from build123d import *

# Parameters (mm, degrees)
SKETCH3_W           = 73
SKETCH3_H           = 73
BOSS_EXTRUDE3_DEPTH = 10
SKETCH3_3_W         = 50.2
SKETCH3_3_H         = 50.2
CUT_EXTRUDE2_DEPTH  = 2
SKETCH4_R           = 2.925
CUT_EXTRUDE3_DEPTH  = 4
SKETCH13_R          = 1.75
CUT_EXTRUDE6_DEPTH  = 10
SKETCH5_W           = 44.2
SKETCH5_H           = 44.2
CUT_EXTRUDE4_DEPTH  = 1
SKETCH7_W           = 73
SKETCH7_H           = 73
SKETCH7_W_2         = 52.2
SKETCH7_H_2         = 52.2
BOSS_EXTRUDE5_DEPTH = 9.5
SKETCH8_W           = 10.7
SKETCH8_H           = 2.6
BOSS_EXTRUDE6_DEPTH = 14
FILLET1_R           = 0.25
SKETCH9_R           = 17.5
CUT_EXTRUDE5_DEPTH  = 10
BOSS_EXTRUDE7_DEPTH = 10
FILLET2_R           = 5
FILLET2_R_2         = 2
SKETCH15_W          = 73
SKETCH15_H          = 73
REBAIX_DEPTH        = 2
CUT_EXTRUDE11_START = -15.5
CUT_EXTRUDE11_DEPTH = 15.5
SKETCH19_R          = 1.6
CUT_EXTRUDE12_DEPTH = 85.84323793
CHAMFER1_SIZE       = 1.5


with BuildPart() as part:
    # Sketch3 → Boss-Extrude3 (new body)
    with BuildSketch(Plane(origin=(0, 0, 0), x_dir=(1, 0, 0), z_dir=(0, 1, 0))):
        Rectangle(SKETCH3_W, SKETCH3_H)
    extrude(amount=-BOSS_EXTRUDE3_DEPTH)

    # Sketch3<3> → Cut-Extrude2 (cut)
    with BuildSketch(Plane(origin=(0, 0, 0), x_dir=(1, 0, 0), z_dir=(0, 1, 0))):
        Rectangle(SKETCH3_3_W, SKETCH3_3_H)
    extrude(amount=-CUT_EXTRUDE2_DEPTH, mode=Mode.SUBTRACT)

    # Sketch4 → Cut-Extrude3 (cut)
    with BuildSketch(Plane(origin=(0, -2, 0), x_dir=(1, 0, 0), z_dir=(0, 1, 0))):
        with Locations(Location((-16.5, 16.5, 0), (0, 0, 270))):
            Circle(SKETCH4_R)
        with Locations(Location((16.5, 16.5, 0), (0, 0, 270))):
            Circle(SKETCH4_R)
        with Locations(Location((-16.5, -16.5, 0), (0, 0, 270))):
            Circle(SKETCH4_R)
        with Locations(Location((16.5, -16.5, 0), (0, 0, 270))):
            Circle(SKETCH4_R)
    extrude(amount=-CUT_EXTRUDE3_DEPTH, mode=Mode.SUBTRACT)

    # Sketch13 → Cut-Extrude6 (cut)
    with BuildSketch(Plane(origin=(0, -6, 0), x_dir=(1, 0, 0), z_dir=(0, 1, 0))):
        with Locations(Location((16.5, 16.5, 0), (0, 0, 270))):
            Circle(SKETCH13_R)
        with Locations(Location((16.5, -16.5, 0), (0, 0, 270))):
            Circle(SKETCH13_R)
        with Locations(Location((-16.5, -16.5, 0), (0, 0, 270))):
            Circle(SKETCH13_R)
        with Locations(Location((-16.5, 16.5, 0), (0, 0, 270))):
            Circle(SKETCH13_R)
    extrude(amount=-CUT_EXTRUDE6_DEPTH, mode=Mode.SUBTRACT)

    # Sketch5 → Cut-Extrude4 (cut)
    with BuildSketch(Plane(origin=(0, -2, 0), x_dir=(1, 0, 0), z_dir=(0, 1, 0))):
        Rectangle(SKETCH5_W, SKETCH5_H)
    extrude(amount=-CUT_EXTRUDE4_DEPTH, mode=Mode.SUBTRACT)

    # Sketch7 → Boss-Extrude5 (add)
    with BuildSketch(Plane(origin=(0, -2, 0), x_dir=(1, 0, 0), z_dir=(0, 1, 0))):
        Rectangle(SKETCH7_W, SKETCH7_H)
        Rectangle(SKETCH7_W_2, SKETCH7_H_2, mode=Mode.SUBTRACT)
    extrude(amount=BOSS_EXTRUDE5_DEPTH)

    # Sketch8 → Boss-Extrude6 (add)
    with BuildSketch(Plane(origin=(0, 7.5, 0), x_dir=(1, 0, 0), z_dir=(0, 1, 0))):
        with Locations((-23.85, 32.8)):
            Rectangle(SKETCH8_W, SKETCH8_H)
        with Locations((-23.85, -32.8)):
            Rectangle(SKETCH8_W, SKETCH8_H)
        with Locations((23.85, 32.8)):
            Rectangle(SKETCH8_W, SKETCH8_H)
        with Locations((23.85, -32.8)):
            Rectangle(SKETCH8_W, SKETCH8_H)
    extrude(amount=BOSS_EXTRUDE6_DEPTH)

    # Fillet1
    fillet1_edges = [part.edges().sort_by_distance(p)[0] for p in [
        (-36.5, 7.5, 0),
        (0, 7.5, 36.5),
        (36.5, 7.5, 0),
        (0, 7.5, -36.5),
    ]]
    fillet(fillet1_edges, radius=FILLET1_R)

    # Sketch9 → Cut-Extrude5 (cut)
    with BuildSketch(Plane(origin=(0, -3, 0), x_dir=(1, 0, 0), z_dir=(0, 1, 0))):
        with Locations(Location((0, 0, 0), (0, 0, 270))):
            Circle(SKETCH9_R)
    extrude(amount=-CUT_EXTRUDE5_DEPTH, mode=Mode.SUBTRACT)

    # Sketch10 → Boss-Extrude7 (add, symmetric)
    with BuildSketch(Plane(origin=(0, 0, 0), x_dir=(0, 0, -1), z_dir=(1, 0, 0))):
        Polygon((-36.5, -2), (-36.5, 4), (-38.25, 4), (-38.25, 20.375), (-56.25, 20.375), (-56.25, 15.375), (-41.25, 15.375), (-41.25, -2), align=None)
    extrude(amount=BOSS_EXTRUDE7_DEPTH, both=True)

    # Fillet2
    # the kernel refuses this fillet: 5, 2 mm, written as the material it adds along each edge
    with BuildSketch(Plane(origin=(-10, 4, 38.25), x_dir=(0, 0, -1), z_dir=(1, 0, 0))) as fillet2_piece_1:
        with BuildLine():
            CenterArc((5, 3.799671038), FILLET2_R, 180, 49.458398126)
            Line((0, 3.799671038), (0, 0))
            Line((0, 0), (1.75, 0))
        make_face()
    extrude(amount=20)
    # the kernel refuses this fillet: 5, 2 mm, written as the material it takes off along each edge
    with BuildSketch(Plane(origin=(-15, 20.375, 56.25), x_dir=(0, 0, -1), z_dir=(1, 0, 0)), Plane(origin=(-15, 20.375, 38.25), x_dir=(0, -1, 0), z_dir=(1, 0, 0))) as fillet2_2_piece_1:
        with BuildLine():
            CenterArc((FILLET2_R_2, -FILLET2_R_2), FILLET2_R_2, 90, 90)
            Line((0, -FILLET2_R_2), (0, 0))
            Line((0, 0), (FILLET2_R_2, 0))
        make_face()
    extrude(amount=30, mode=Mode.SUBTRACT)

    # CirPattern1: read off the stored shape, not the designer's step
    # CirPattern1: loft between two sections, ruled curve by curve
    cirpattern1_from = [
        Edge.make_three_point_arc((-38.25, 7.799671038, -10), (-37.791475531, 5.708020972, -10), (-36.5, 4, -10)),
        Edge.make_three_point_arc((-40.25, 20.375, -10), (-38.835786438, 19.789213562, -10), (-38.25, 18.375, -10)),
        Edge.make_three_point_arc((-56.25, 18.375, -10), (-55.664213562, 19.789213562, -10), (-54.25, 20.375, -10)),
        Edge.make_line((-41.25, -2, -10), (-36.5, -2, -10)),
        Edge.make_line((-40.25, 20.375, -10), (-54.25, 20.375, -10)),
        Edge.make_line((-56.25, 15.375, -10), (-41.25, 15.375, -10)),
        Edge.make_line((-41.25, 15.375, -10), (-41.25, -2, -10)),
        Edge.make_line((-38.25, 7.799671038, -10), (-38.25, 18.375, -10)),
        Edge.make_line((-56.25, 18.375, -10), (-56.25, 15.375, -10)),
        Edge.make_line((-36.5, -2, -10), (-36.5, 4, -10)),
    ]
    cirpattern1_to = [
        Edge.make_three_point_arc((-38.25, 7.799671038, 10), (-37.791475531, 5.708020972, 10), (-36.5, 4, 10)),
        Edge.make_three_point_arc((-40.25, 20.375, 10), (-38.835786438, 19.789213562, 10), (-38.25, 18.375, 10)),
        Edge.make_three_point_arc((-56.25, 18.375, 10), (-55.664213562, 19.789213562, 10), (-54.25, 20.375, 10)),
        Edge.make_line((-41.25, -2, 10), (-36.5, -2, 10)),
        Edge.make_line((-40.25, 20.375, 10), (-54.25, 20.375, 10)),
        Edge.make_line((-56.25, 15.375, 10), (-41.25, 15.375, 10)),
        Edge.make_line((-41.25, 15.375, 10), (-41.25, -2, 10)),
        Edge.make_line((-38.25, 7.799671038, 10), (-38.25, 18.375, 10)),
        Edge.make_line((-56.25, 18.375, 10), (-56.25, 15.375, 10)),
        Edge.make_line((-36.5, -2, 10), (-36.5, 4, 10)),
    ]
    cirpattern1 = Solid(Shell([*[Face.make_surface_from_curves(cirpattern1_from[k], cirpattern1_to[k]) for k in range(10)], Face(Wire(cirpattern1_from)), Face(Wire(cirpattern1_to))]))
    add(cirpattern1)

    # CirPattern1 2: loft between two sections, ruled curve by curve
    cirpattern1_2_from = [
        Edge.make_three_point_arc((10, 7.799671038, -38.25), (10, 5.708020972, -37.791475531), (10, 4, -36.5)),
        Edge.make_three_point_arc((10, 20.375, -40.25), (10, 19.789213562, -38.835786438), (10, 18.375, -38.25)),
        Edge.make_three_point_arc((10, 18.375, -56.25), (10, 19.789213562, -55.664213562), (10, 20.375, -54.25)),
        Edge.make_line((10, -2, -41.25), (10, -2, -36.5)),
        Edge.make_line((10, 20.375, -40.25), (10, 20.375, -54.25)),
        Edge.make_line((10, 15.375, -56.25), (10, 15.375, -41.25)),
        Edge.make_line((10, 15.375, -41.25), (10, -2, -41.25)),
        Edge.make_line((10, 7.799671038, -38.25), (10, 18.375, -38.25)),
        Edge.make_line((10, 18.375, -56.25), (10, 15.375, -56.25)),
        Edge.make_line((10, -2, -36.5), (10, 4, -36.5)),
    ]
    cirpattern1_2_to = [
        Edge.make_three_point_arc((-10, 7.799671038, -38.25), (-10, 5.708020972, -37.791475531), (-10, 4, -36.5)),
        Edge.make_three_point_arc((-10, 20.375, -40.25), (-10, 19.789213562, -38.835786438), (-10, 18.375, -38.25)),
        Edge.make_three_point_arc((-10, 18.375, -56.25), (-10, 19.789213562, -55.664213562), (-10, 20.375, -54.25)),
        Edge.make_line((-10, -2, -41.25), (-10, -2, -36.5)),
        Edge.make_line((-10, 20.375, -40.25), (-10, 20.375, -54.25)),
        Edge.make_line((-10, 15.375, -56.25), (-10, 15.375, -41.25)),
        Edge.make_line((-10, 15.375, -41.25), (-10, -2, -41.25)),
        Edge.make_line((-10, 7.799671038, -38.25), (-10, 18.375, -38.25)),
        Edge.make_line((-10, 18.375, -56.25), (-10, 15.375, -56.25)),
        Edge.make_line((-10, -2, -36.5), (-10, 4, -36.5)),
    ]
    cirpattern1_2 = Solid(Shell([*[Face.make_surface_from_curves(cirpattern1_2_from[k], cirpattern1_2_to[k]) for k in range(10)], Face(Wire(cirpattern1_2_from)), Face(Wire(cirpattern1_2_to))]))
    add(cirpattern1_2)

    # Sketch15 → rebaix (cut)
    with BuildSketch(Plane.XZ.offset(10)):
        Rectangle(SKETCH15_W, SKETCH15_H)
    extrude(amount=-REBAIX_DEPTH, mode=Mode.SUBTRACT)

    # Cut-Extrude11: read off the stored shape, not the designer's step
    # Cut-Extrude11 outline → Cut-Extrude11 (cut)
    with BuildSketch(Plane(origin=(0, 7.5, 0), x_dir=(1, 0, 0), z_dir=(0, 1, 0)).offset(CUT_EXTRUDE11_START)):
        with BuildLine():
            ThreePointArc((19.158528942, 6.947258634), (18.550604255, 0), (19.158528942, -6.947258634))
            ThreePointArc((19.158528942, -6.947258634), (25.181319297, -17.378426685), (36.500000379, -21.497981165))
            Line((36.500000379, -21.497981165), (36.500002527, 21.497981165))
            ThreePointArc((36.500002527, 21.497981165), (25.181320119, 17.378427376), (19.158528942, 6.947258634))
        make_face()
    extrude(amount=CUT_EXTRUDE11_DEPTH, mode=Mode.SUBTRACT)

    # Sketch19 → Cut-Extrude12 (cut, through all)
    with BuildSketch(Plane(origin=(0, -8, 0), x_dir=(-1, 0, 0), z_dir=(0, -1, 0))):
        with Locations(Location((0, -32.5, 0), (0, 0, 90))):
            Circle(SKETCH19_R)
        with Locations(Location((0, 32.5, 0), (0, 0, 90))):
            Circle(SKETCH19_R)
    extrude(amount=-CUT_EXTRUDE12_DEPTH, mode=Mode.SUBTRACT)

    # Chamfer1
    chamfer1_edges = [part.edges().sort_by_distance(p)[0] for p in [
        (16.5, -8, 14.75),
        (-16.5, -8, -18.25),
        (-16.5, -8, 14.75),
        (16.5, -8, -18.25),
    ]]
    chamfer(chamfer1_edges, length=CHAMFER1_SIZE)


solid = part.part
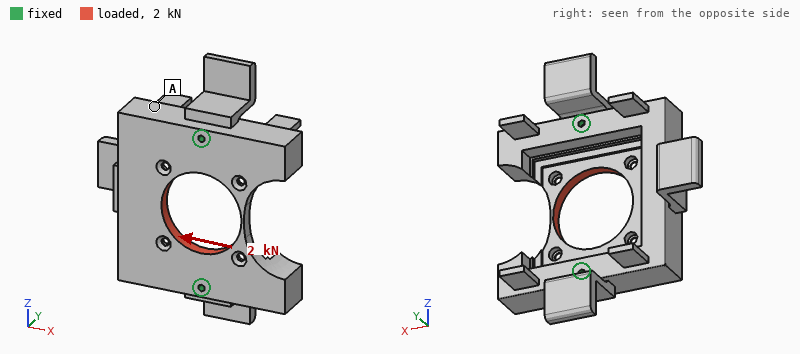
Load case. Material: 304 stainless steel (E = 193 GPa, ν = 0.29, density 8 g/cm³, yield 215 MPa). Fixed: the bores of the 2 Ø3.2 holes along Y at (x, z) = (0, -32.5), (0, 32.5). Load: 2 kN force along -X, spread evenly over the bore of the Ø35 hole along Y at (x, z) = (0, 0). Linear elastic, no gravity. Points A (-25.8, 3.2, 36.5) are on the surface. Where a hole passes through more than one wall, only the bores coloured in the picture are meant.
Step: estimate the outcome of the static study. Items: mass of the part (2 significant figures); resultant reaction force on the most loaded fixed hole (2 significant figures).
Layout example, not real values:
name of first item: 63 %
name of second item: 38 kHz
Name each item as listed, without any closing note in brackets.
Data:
mass of the part: 420 g
resultant reaction force on the most loaded fixed hole: 1.0 kN
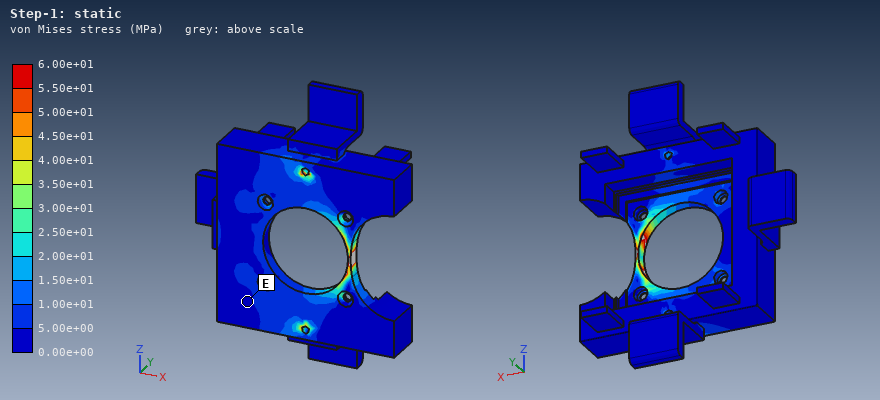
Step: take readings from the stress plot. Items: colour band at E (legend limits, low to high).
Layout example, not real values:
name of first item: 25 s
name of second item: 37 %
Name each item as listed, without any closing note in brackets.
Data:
colour band at E: 0.00e+00 to 5.00e+00 MPa
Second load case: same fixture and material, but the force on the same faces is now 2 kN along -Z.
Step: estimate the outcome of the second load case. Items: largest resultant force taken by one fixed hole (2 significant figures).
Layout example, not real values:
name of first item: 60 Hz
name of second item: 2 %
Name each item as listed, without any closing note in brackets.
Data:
largest resultant force taken by one fixed hole: 1.0 kN
